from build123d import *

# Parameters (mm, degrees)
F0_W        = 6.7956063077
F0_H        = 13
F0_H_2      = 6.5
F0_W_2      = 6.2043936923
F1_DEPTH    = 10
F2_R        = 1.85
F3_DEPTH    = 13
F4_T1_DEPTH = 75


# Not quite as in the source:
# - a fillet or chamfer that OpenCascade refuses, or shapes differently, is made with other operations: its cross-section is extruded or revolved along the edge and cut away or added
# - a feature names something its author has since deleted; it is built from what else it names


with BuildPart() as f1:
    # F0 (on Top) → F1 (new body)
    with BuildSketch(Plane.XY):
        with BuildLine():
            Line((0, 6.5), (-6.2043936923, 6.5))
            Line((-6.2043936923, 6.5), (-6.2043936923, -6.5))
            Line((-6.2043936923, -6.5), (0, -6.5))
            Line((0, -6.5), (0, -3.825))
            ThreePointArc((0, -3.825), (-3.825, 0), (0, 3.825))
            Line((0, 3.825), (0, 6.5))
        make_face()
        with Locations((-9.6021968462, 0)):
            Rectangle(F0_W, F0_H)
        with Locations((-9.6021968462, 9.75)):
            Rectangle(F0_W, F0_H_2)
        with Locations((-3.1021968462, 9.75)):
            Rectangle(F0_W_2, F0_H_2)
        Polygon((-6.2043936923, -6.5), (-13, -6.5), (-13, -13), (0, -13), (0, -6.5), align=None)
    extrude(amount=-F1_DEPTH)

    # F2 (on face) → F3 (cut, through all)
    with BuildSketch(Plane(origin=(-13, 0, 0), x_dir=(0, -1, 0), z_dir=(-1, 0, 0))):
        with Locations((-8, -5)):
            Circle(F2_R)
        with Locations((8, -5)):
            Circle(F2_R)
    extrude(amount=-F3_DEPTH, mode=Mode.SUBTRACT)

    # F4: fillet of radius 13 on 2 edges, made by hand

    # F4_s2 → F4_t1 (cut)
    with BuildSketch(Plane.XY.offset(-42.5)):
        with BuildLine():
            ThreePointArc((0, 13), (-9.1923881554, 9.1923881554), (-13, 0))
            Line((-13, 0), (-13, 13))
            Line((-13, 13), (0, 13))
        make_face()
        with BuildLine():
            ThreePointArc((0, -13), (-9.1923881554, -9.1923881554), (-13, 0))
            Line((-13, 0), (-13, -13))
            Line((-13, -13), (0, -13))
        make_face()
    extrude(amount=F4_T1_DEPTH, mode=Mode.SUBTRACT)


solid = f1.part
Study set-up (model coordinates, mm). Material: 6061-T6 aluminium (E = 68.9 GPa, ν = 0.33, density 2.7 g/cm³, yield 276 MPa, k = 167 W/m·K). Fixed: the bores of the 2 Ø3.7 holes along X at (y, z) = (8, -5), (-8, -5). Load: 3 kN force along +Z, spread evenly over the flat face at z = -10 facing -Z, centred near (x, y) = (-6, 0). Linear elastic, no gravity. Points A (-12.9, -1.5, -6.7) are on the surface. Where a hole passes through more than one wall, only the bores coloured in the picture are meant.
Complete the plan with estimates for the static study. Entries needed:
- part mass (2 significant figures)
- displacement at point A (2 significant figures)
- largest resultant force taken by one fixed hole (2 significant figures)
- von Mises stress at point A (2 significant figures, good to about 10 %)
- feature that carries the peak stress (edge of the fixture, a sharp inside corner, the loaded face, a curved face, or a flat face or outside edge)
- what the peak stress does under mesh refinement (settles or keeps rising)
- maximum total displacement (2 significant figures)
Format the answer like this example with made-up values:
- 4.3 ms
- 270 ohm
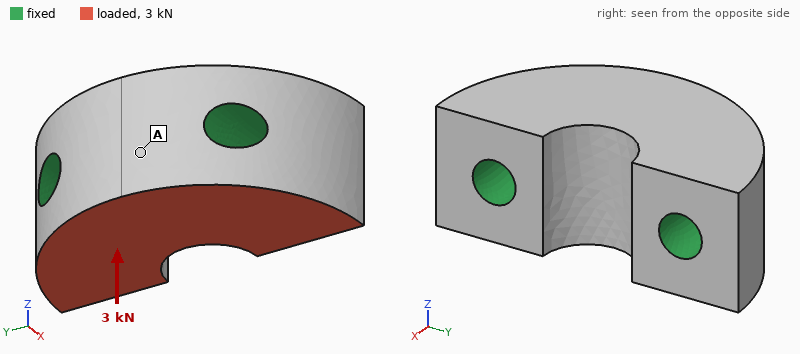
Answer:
- 6.0 g
- 2.6 µm
- 1.5 kN
- 9.3 MPa
- edge of the fixture
- keeps rising
- 3.4 µm
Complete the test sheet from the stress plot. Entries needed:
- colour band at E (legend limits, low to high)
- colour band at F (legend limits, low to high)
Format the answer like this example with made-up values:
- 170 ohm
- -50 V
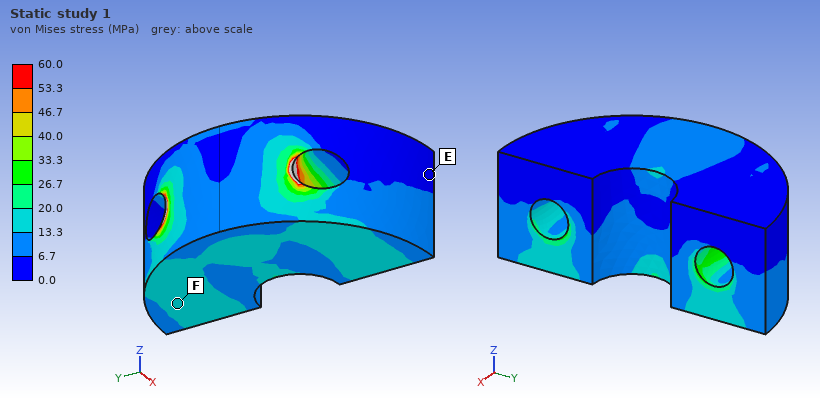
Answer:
- 0.0 to 6.7 MPa
- 13.3 to 20.0 MPa
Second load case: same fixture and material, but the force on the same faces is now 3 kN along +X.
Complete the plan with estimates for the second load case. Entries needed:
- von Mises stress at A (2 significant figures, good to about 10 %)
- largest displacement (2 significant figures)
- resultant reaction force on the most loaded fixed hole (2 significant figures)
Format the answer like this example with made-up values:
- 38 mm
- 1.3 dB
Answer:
- 20 MPa
- 7.6 µm
- 1.5 kN
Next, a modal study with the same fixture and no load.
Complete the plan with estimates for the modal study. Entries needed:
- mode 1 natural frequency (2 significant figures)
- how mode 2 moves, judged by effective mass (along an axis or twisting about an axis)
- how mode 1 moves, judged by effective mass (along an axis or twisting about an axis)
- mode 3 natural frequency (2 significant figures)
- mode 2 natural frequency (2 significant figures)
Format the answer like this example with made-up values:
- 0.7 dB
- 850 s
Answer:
- 79 kHz
- along X
- along Z
- 110 kHz
- 95 kHz
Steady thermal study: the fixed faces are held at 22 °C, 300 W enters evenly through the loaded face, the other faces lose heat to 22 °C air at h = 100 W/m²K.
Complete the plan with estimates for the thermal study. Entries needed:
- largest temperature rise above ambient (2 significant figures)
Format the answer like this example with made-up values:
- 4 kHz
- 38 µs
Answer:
- 49 K
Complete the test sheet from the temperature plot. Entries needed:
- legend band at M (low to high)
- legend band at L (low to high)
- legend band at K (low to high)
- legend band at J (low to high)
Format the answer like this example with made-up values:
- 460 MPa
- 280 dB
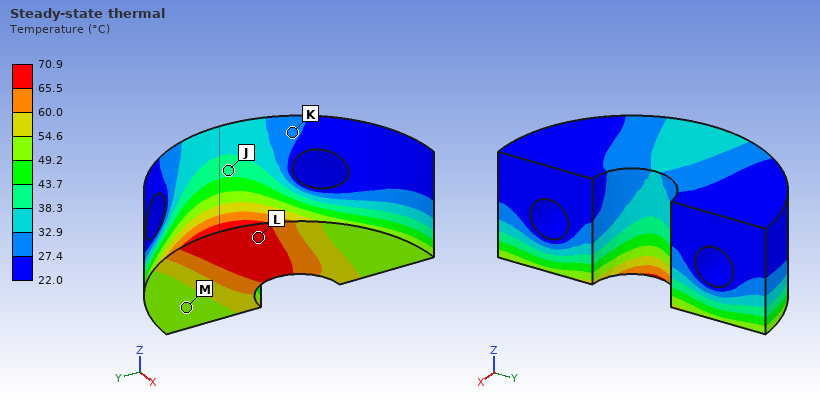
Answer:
- 49.2 to 54.6 °C
- 65.5 to 70.9 °C
- 27.4 to 32.9 °C
- 38.3 to 43.7 °C
